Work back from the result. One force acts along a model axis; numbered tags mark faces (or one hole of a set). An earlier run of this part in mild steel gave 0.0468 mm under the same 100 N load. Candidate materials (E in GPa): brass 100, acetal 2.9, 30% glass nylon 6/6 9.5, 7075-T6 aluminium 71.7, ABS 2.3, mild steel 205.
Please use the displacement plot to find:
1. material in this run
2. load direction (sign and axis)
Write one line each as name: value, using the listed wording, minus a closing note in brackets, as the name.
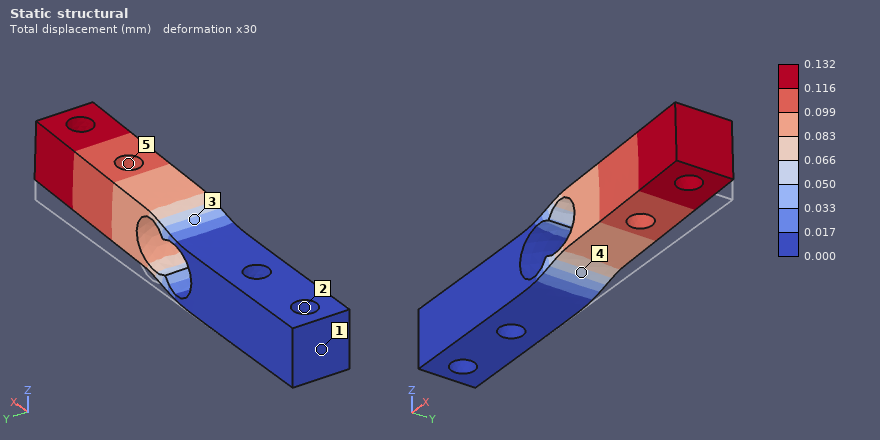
material in this run: 7075-T6 aluminium
load direction: +Z
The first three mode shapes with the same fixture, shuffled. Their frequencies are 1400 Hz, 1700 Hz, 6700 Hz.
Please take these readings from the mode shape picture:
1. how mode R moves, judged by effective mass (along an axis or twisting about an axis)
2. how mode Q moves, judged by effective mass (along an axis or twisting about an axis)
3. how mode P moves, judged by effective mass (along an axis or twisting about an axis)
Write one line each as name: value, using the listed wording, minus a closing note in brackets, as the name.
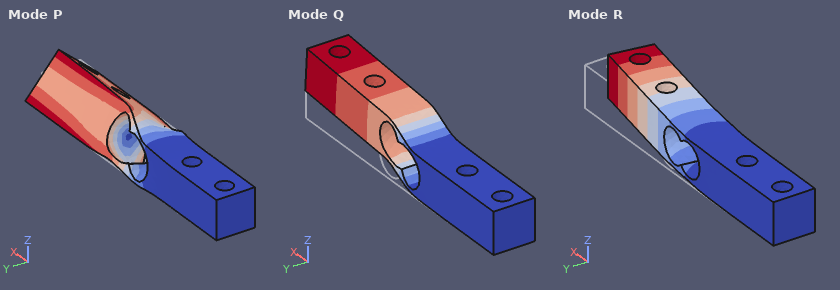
how mode R moves, judged by effective mass: along Y
how mode Q moves, judged by effective mass: along Z
how mode P moves, judged by effective mass: twisting about X
